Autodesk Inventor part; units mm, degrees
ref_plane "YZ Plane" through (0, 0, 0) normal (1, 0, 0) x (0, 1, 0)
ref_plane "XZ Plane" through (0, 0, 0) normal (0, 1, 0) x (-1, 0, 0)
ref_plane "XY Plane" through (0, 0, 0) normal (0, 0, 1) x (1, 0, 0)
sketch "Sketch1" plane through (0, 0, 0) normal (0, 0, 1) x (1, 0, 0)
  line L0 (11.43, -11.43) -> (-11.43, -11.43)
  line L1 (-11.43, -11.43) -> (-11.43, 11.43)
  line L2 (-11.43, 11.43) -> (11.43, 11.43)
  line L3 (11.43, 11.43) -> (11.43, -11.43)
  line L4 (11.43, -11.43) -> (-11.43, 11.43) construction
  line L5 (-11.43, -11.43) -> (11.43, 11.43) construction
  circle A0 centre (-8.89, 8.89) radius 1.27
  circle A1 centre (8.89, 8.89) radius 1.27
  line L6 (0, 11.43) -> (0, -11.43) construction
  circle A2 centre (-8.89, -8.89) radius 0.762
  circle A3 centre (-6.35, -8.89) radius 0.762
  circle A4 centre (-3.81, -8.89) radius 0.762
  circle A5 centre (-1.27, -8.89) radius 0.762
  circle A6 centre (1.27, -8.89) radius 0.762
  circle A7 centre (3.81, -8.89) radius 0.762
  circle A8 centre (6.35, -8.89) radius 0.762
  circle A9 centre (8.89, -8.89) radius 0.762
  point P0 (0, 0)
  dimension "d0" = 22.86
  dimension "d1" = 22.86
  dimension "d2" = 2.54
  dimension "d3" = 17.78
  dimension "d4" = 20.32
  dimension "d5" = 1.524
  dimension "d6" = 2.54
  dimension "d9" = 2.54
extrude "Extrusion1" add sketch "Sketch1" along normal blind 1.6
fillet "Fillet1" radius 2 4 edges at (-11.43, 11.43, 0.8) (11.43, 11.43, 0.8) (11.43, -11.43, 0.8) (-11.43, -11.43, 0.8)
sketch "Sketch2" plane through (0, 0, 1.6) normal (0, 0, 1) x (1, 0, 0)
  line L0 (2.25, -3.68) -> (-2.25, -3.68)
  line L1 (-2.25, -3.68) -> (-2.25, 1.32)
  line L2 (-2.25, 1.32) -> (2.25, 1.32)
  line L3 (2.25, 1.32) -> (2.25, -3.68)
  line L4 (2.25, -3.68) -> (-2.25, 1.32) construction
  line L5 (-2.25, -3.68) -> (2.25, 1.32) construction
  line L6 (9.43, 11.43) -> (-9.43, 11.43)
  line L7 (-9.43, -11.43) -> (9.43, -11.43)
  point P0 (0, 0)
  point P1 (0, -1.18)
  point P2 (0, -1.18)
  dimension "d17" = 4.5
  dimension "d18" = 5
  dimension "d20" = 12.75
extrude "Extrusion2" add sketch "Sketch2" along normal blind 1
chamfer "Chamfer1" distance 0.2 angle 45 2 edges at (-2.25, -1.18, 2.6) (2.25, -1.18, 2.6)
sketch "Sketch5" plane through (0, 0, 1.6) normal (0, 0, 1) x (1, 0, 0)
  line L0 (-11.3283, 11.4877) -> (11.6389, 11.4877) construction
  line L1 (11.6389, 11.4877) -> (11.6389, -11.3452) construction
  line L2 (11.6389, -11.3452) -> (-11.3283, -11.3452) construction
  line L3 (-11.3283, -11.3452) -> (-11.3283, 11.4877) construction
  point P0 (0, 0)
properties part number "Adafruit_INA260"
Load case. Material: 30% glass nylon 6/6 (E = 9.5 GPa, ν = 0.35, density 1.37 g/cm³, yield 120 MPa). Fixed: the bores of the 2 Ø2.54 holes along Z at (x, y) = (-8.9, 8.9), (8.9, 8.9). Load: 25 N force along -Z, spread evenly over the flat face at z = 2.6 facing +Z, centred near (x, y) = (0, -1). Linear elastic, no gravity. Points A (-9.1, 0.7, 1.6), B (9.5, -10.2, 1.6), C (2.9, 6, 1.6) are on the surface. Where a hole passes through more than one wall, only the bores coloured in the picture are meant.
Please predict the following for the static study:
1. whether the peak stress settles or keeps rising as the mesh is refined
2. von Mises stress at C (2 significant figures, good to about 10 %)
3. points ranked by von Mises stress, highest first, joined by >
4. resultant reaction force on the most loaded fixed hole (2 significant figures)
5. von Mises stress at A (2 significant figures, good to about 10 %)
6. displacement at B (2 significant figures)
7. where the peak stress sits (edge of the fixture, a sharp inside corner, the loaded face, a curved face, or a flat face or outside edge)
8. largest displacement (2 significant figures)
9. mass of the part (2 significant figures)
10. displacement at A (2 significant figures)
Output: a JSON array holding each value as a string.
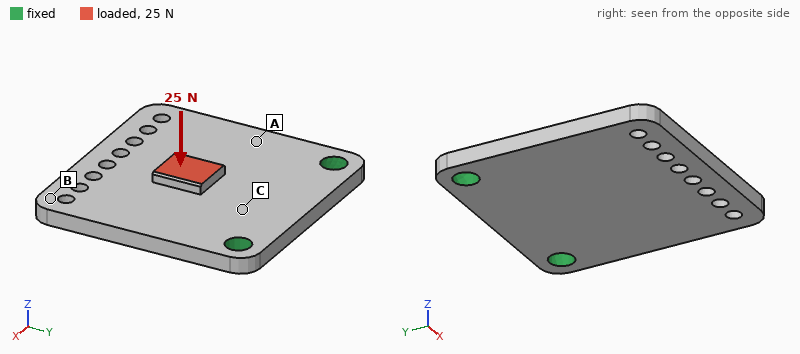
["keeps rising", "12 MPa", "C > A > B", "13 N", "7.4 MPa", "0.30 mm", "edge of the fixture", "0.35 mm", "1.1 g", "0.083 mm"]
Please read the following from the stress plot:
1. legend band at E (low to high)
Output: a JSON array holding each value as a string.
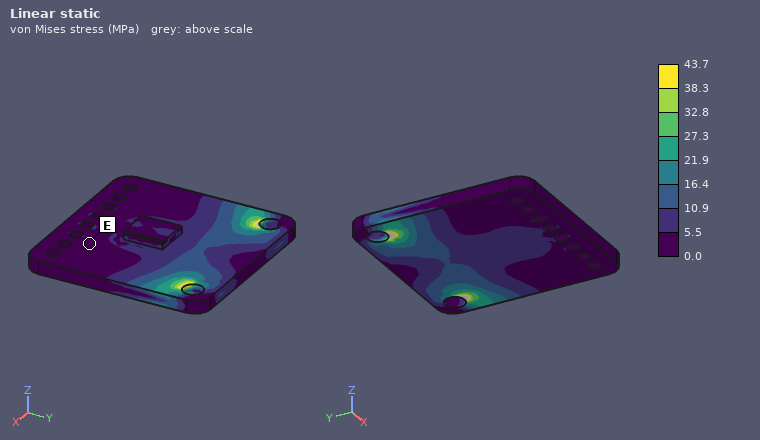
["0.0 to 5.5 MPa"]
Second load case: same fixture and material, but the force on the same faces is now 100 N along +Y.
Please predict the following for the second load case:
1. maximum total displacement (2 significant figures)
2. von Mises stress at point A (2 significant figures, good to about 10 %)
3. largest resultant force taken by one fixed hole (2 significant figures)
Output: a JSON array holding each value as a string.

["0.38 mm", "14 MPa", "54 N"]
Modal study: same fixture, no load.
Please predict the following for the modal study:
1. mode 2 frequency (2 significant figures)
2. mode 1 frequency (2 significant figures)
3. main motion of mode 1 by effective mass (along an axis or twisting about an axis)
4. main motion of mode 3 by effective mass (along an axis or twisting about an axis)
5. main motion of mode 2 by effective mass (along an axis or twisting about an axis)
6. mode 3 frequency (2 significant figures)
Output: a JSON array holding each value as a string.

["4100 Hz", "1700 Hz", "along Z", "along Z", "twisting about Y", "10 kHz"]
